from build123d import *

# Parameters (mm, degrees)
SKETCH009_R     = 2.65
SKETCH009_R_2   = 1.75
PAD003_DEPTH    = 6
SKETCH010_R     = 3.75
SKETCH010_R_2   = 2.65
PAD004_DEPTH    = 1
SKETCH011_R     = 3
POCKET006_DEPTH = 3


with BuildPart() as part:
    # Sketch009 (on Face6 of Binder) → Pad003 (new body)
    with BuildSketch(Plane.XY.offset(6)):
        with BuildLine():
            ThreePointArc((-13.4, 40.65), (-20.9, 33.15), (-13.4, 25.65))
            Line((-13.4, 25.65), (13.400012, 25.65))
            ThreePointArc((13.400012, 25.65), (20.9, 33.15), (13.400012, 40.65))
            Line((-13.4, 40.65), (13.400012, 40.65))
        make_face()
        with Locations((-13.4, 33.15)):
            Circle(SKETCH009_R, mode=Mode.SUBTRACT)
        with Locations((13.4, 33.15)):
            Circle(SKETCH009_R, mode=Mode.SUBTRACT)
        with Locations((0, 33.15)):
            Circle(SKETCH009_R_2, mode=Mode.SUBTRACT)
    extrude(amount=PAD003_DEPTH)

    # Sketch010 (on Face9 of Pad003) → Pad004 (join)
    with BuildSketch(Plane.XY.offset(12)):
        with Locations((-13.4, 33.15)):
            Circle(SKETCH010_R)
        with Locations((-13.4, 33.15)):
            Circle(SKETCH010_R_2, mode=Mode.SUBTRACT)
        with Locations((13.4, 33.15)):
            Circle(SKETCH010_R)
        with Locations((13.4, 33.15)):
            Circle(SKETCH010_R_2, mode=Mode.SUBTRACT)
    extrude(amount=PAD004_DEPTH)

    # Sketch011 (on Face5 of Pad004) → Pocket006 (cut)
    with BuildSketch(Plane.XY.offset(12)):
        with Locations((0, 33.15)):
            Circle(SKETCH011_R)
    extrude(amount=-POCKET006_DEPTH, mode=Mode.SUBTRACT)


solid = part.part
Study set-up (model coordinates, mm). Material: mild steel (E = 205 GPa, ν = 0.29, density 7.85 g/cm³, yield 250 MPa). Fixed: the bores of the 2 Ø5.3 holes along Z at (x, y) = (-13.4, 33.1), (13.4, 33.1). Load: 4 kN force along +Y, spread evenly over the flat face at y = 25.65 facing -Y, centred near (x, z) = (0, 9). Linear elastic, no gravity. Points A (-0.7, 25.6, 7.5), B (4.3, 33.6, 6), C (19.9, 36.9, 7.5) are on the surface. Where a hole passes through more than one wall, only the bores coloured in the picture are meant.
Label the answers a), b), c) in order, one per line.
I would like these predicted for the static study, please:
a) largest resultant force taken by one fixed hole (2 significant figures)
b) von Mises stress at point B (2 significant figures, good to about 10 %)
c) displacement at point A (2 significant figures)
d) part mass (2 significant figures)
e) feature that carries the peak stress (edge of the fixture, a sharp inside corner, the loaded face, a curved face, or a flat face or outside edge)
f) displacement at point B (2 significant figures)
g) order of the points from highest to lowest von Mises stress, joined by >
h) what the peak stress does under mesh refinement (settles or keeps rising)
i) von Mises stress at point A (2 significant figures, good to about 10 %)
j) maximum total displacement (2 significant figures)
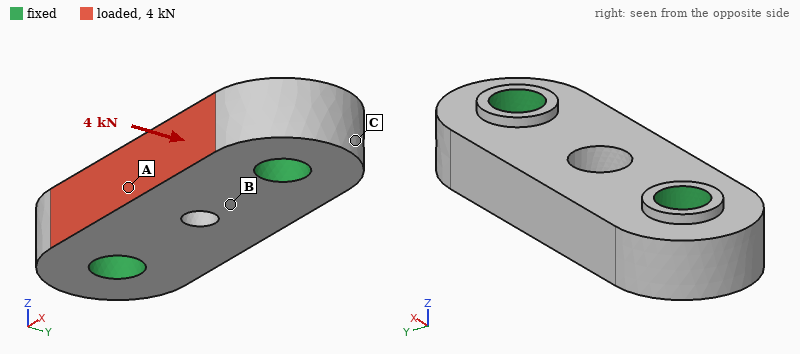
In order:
a) 2.0 kN
b) 22 MPa
c) 3.3 µm
d) 25 g
e) edge of the fixture
f) 2.2 µm
g) A > B > C
h) keeps rising
i) 41 MPa
j) 3.5 µm
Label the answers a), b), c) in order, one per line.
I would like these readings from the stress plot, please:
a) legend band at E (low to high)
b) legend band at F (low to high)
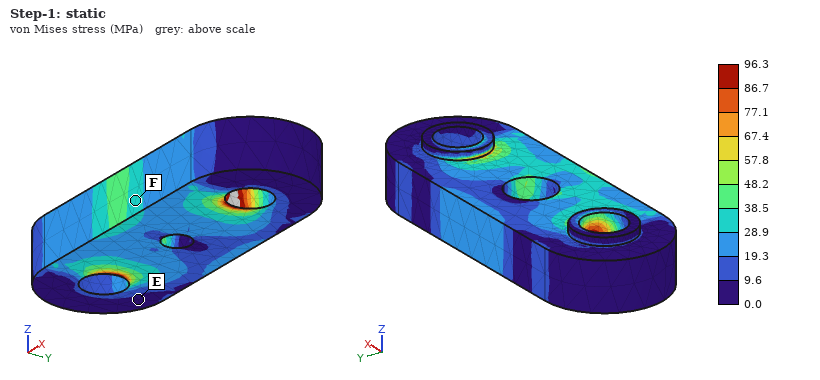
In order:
a) 0.0 to 9.6 MPa
b) 28.9 to 38.5 MPa
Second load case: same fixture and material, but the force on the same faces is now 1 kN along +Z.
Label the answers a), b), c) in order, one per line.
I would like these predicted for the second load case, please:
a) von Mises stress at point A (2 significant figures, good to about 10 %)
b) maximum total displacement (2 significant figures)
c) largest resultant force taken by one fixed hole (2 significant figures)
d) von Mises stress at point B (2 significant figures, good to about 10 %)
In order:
a) 16 MPa
b) 4.4 µm
c) 500 N
d) 18 MPa
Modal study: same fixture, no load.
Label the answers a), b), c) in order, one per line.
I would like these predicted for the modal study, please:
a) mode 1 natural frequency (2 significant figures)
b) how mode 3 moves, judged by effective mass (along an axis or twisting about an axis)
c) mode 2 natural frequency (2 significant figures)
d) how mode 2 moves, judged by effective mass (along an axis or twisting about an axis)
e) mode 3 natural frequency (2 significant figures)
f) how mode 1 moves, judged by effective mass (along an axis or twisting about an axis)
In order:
a) 40 kHz
b) along Y
c) 45 kHz
d) twisting about X
e) 52 kHz
f) along Z
